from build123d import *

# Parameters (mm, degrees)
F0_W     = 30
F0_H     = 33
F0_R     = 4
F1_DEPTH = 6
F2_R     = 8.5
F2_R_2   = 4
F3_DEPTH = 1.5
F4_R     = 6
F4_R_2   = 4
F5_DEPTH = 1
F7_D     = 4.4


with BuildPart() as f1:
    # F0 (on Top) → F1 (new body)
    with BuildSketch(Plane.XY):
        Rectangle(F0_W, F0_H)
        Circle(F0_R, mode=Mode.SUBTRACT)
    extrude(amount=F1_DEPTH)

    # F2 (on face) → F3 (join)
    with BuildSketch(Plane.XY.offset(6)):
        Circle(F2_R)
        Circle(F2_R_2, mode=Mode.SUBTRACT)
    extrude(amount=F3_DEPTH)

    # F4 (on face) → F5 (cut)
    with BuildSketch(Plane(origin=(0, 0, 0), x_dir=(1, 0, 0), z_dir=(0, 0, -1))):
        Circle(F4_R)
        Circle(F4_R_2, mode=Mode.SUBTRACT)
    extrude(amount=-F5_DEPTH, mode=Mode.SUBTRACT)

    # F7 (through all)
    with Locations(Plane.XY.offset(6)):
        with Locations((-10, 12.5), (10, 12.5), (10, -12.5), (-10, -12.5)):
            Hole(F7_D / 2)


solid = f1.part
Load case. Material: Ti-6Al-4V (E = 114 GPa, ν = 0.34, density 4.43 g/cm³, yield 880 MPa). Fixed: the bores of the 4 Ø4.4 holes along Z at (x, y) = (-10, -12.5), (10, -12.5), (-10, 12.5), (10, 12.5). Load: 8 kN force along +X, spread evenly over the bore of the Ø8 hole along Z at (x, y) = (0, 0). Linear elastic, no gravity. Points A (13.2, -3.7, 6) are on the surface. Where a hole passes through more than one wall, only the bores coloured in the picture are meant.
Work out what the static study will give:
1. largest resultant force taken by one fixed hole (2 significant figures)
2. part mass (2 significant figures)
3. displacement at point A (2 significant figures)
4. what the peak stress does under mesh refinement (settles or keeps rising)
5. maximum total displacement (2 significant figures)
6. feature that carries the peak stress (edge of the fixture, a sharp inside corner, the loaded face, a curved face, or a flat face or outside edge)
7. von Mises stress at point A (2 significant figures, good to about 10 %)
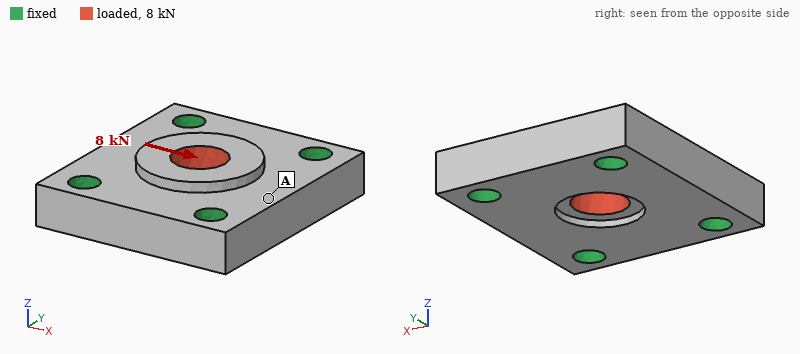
2.2 kN
24 g
4.8 µm
keeps rising
8.4 µm
edge of the fixture
19 MPa
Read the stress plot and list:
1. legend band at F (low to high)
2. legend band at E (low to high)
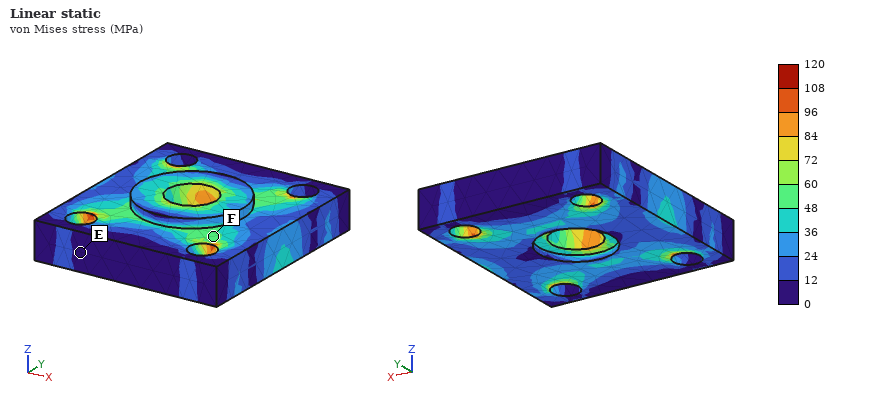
48 to 60 MPa
0 to 12 MPa
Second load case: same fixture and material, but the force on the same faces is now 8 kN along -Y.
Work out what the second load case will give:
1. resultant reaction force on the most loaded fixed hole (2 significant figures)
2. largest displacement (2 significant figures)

2.2 kN
6.6 µm
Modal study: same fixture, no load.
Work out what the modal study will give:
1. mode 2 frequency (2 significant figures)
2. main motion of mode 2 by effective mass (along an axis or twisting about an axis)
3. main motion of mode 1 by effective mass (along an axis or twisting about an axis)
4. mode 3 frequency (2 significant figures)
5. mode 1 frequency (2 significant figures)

46 kHz
twisting about Y
along Z
56 kHz
39 kHz
